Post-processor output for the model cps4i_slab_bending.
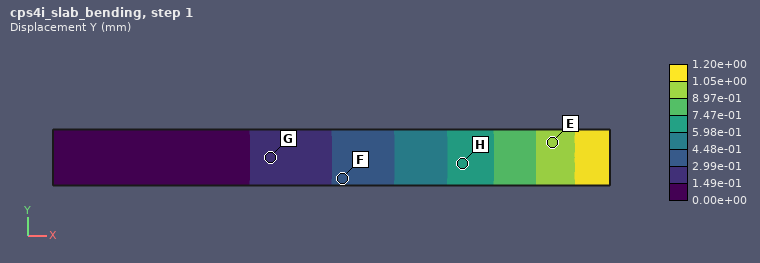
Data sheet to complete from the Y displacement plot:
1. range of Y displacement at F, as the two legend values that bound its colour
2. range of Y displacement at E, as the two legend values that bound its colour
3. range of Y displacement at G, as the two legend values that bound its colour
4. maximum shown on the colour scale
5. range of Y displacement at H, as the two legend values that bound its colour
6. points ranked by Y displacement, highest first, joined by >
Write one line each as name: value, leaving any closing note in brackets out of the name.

range of Y displacement at F, as the two legend values that bound its colour: 2.99e-01 to 4.48e-01 mm
range of Y displacement at E, as the two legend values that bound its colour: 8.97e-01 to 1.05e+00 mm
range of Y displacement at G, as the two legend values that bound its colour: 1.49e-01 to 2.99e-01 mm
maximum shown on the colour scale: 1.20e+00 mm
range of Y displacement at H, as the two legend values that bound its colour: 5.98e-01 to 7.47e-01 mm
points ranked by Y displacement, highest first, joined by >: E > H > F > G
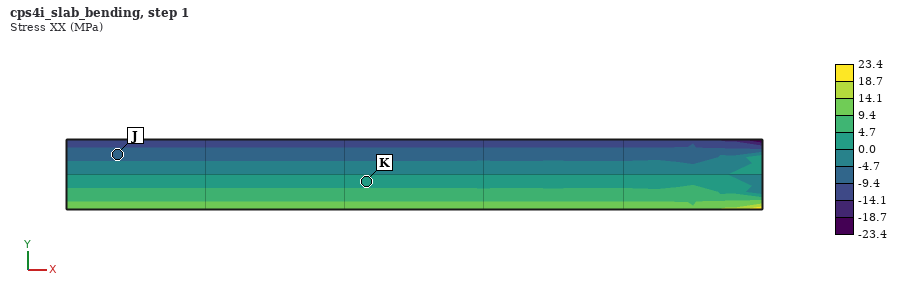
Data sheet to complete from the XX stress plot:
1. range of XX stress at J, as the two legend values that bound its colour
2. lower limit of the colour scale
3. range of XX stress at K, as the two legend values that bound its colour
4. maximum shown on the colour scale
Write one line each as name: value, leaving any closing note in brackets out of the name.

range of XX stress at J, as the two legend values that bound its colour: -9.4 to -4.7 MPa
lower limit of the colour scale: -23.4 MPa
range of XX stress at K, as the two legend values that bound its colour: 0.0 to 4.7 MPa
maximum shown on the colour scale: 23.4 MPa
